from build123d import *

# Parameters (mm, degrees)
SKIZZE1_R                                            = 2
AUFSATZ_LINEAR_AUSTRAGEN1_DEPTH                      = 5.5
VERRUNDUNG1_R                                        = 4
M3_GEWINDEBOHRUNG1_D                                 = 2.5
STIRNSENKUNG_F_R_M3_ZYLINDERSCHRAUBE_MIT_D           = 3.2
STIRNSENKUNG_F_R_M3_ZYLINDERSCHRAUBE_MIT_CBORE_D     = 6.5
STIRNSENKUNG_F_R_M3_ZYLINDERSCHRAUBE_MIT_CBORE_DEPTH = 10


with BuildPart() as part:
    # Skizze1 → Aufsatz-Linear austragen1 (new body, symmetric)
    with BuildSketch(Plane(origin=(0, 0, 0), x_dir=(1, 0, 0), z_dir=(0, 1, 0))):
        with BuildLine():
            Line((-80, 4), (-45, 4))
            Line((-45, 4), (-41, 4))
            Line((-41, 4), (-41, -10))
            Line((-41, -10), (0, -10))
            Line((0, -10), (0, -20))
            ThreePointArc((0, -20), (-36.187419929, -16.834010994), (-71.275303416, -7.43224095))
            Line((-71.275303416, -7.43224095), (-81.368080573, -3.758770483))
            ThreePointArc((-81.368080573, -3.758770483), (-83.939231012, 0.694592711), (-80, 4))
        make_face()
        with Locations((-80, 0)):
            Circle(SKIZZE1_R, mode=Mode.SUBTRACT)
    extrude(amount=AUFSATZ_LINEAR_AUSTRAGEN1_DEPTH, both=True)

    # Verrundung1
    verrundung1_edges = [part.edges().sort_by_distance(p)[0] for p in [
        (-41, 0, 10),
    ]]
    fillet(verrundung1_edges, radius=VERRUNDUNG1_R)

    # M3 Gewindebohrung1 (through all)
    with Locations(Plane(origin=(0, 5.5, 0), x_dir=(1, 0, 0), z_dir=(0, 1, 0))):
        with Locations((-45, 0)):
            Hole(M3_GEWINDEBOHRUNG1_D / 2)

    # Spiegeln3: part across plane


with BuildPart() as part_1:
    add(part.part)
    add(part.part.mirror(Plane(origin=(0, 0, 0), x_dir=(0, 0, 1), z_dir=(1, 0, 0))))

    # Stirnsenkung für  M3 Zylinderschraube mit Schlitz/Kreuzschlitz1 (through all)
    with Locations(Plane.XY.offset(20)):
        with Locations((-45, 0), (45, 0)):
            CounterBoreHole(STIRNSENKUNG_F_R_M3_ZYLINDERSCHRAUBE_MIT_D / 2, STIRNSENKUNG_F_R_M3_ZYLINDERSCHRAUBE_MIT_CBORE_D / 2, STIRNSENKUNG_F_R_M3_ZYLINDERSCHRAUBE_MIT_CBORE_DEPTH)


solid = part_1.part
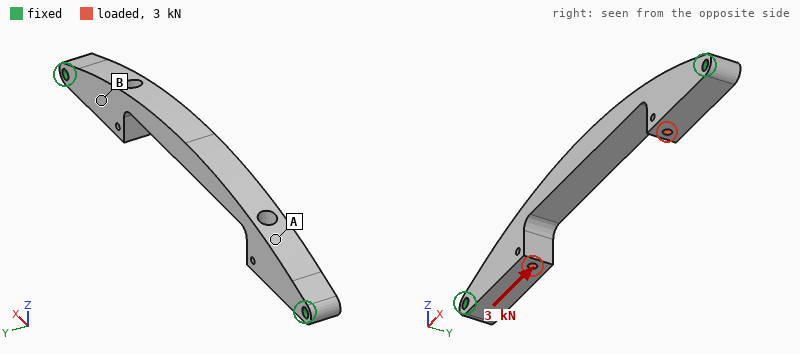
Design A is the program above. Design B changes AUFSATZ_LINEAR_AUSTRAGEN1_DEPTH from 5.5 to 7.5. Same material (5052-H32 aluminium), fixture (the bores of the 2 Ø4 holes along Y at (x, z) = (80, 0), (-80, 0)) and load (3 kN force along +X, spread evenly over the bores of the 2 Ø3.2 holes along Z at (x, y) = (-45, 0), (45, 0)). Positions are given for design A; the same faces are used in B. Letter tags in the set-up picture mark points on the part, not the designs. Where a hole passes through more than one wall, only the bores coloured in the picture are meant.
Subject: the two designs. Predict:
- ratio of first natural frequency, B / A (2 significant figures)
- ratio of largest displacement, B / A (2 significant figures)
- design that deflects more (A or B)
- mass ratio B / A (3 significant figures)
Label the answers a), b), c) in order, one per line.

a) 1.3
b) 0.72
c) A
d) 1.37
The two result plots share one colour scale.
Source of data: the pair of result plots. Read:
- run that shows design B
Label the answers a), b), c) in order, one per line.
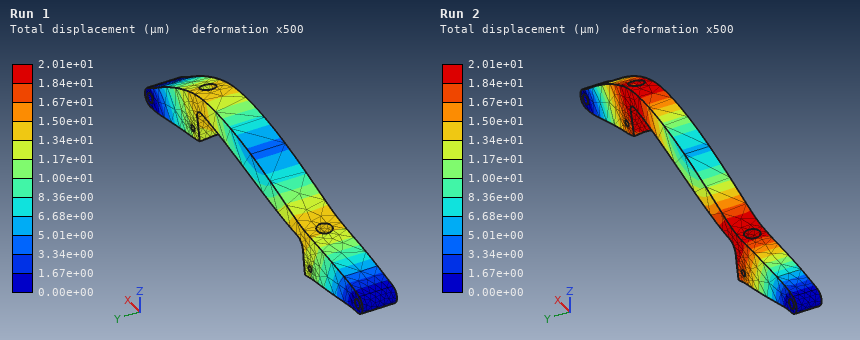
a) Run 1
